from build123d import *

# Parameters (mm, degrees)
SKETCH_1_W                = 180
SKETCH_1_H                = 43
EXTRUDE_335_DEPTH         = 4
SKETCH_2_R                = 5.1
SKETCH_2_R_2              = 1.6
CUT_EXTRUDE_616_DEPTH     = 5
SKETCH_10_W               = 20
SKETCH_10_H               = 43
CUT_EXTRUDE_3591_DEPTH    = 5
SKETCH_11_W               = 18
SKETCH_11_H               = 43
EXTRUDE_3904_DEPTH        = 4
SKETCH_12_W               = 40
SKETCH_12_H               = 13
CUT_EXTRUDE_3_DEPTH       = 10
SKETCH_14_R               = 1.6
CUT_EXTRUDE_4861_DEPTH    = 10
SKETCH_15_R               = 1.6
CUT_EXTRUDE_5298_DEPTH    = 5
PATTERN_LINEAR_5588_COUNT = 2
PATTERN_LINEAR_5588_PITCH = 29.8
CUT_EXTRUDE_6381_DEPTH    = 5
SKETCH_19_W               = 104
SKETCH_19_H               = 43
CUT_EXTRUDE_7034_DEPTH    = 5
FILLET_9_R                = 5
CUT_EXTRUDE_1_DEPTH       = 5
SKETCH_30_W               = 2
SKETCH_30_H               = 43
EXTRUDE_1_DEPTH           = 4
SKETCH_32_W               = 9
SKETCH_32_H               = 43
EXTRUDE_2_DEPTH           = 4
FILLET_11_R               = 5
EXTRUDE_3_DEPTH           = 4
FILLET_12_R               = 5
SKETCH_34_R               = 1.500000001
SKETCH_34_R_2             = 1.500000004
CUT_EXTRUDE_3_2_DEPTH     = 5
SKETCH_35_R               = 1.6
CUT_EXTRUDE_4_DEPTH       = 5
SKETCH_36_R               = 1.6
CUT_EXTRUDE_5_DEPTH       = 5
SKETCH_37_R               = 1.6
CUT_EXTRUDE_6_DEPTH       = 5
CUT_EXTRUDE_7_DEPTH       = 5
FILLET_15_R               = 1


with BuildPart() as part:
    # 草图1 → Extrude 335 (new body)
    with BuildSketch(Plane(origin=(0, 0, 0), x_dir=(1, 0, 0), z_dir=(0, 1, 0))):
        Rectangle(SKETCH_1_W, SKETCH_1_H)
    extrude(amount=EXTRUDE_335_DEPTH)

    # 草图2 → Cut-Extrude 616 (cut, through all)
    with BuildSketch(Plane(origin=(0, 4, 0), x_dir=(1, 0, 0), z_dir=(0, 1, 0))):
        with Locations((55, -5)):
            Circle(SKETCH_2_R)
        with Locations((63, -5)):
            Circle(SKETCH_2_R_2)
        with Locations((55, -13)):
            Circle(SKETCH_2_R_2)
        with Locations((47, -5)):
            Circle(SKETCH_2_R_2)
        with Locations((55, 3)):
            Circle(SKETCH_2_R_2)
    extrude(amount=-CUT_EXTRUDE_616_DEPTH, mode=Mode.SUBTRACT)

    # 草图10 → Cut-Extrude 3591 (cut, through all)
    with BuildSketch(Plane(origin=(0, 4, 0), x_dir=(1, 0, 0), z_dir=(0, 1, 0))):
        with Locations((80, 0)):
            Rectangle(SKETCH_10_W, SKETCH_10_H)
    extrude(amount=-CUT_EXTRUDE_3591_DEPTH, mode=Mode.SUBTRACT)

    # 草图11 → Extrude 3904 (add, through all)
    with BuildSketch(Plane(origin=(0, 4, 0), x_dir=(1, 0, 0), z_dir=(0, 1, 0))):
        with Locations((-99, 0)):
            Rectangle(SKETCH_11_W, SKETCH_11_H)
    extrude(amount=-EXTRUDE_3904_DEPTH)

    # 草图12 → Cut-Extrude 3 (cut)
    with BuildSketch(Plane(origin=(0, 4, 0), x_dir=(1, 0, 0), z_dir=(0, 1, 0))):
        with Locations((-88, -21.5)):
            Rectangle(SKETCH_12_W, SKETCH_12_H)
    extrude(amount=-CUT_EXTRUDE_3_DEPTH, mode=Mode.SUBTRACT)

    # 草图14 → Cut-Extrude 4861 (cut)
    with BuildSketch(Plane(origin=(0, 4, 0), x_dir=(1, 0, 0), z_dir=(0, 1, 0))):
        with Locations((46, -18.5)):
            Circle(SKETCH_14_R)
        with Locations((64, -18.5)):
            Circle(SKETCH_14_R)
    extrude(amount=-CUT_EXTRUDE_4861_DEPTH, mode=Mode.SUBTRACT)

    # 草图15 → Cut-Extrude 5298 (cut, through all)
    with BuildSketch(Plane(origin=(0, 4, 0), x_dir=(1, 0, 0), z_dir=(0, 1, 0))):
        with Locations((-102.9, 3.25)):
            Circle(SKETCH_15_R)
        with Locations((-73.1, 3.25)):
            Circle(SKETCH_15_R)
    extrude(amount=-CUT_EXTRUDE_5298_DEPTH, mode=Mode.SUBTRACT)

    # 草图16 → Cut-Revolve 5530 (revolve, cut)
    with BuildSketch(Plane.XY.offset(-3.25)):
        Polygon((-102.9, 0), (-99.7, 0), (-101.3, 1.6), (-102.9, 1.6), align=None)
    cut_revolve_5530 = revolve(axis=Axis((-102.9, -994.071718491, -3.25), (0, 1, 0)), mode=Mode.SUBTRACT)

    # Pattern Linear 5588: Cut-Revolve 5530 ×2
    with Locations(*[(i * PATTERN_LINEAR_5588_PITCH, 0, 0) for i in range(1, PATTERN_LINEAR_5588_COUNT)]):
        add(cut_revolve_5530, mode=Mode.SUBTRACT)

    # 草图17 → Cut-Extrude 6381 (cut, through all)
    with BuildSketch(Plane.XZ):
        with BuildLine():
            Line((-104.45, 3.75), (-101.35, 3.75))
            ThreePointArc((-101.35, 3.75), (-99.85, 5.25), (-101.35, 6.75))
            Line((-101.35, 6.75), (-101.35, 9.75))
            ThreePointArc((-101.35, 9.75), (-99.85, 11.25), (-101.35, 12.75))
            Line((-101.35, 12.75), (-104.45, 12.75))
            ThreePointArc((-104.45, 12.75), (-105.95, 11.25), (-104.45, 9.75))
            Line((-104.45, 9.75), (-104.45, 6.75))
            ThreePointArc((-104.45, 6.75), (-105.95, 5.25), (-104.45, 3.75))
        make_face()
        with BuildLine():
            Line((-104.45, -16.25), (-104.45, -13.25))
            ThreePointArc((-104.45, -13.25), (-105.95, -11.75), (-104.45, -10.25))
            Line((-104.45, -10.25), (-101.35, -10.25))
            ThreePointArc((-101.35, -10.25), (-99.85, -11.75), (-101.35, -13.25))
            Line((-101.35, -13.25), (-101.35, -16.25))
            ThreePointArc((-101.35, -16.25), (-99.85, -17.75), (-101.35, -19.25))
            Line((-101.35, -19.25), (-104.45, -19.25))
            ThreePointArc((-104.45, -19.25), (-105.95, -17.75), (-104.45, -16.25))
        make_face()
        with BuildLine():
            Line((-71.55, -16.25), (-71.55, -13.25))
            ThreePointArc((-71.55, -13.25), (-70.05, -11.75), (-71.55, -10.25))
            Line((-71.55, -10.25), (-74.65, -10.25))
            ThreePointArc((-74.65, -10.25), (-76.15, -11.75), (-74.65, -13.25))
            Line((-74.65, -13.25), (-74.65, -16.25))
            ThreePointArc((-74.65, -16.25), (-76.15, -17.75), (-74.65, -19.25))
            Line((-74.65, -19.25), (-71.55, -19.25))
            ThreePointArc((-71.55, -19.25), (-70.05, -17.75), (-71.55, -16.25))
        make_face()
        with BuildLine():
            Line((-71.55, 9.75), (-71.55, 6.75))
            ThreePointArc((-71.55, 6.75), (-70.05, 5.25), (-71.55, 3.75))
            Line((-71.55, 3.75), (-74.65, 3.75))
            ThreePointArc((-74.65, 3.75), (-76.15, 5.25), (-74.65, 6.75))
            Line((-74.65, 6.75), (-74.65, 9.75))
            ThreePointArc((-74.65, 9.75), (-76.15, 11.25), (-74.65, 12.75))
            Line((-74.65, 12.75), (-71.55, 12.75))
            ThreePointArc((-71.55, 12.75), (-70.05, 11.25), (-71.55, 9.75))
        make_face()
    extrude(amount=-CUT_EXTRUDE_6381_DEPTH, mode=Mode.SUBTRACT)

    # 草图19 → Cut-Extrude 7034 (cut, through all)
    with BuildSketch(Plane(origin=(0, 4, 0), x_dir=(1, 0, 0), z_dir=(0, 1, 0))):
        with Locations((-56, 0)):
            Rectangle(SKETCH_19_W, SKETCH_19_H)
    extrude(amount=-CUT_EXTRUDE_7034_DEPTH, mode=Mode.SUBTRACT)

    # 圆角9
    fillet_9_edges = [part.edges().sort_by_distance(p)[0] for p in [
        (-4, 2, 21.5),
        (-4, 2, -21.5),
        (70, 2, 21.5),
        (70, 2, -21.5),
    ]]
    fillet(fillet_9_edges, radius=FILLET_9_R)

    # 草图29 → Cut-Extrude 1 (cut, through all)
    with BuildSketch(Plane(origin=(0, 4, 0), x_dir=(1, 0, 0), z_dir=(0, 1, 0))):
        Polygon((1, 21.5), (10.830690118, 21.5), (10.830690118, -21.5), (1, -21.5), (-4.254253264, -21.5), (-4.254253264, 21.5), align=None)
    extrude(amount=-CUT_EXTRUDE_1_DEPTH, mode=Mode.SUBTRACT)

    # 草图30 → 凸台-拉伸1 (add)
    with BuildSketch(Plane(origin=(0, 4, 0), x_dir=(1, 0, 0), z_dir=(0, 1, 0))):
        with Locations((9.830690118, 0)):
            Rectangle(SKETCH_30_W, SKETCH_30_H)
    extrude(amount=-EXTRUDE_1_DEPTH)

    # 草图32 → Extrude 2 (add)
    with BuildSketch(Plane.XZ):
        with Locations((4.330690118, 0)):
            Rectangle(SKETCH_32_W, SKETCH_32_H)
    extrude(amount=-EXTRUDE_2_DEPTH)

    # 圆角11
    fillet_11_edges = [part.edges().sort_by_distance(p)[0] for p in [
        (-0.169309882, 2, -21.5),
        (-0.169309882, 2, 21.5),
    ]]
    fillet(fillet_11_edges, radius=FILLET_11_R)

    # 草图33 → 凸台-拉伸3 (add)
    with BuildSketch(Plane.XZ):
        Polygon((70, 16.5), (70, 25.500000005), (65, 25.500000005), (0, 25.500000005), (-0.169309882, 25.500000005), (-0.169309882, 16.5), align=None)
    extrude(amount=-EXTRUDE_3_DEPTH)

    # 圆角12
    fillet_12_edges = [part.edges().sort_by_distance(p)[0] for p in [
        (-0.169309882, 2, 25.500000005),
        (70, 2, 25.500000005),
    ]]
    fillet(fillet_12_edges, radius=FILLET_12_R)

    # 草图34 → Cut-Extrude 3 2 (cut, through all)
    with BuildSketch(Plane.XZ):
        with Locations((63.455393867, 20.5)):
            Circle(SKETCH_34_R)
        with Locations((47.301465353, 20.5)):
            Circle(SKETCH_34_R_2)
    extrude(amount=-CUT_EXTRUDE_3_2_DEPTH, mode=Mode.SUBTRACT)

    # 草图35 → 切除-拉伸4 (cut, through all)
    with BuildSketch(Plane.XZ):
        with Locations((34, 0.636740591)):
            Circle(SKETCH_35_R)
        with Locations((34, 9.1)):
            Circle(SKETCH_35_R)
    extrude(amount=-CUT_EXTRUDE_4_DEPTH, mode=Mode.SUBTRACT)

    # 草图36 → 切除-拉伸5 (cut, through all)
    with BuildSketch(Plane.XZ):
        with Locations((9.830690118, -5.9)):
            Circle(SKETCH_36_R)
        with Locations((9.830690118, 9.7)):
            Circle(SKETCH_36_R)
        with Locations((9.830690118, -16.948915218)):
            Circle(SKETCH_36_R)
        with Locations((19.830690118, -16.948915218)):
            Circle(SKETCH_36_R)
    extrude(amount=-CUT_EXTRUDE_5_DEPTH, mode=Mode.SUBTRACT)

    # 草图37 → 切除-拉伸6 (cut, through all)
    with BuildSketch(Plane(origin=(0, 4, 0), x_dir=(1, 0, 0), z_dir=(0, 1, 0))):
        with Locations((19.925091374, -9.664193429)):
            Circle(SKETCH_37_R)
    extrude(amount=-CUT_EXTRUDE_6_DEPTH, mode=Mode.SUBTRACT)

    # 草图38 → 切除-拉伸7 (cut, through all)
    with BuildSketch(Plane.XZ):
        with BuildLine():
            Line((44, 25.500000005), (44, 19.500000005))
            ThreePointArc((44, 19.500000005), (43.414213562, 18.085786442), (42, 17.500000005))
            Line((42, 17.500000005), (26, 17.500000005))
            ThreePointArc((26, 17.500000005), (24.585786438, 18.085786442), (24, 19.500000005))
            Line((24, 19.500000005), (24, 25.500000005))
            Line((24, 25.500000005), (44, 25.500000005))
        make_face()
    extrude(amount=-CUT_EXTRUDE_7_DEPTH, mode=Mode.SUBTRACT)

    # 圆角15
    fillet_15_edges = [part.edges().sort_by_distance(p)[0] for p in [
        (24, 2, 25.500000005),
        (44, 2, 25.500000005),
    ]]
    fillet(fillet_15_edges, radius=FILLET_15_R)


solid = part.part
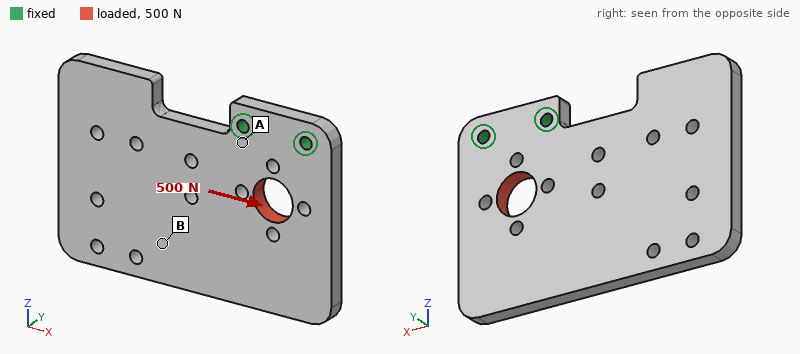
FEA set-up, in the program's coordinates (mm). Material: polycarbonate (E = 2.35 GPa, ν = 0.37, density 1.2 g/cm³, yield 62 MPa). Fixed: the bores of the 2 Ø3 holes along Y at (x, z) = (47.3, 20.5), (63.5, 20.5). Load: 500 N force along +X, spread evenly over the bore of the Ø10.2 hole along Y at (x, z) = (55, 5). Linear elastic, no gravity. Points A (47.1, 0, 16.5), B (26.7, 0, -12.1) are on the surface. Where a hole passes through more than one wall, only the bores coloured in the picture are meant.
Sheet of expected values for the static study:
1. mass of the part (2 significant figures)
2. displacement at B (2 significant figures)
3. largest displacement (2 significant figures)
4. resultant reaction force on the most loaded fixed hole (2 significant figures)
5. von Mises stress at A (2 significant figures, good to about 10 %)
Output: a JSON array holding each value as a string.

["14 g", "0.47 mm", "0.73 mm", "480 N", "15 MPa"]
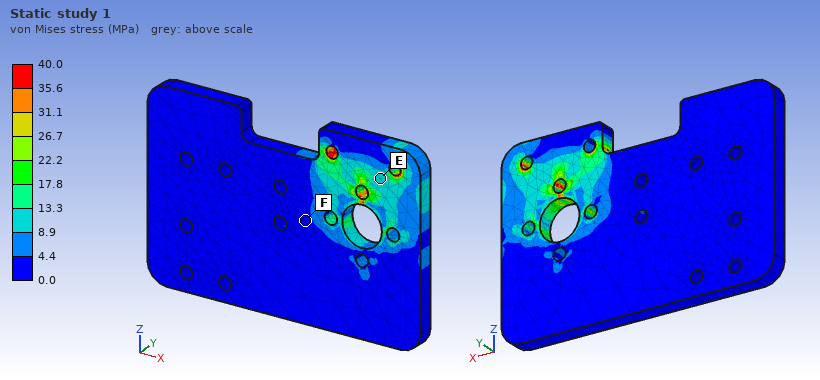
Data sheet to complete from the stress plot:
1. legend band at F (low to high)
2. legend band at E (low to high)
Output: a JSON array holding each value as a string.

["0.0 to 4.4 MPa", "8.9 to 13.3 MPa"]
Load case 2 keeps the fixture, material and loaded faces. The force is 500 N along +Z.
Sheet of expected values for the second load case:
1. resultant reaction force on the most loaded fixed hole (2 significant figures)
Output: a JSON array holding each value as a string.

["260 N"]
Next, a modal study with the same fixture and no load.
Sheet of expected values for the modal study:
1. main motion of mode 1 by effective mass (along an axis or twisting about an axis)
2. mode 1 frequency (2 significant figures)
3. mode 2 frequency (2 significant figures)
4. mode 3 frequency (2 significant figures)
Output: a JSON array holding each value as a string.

["along Y", "210 Hz", "380 Hz", "870 Hz"]
